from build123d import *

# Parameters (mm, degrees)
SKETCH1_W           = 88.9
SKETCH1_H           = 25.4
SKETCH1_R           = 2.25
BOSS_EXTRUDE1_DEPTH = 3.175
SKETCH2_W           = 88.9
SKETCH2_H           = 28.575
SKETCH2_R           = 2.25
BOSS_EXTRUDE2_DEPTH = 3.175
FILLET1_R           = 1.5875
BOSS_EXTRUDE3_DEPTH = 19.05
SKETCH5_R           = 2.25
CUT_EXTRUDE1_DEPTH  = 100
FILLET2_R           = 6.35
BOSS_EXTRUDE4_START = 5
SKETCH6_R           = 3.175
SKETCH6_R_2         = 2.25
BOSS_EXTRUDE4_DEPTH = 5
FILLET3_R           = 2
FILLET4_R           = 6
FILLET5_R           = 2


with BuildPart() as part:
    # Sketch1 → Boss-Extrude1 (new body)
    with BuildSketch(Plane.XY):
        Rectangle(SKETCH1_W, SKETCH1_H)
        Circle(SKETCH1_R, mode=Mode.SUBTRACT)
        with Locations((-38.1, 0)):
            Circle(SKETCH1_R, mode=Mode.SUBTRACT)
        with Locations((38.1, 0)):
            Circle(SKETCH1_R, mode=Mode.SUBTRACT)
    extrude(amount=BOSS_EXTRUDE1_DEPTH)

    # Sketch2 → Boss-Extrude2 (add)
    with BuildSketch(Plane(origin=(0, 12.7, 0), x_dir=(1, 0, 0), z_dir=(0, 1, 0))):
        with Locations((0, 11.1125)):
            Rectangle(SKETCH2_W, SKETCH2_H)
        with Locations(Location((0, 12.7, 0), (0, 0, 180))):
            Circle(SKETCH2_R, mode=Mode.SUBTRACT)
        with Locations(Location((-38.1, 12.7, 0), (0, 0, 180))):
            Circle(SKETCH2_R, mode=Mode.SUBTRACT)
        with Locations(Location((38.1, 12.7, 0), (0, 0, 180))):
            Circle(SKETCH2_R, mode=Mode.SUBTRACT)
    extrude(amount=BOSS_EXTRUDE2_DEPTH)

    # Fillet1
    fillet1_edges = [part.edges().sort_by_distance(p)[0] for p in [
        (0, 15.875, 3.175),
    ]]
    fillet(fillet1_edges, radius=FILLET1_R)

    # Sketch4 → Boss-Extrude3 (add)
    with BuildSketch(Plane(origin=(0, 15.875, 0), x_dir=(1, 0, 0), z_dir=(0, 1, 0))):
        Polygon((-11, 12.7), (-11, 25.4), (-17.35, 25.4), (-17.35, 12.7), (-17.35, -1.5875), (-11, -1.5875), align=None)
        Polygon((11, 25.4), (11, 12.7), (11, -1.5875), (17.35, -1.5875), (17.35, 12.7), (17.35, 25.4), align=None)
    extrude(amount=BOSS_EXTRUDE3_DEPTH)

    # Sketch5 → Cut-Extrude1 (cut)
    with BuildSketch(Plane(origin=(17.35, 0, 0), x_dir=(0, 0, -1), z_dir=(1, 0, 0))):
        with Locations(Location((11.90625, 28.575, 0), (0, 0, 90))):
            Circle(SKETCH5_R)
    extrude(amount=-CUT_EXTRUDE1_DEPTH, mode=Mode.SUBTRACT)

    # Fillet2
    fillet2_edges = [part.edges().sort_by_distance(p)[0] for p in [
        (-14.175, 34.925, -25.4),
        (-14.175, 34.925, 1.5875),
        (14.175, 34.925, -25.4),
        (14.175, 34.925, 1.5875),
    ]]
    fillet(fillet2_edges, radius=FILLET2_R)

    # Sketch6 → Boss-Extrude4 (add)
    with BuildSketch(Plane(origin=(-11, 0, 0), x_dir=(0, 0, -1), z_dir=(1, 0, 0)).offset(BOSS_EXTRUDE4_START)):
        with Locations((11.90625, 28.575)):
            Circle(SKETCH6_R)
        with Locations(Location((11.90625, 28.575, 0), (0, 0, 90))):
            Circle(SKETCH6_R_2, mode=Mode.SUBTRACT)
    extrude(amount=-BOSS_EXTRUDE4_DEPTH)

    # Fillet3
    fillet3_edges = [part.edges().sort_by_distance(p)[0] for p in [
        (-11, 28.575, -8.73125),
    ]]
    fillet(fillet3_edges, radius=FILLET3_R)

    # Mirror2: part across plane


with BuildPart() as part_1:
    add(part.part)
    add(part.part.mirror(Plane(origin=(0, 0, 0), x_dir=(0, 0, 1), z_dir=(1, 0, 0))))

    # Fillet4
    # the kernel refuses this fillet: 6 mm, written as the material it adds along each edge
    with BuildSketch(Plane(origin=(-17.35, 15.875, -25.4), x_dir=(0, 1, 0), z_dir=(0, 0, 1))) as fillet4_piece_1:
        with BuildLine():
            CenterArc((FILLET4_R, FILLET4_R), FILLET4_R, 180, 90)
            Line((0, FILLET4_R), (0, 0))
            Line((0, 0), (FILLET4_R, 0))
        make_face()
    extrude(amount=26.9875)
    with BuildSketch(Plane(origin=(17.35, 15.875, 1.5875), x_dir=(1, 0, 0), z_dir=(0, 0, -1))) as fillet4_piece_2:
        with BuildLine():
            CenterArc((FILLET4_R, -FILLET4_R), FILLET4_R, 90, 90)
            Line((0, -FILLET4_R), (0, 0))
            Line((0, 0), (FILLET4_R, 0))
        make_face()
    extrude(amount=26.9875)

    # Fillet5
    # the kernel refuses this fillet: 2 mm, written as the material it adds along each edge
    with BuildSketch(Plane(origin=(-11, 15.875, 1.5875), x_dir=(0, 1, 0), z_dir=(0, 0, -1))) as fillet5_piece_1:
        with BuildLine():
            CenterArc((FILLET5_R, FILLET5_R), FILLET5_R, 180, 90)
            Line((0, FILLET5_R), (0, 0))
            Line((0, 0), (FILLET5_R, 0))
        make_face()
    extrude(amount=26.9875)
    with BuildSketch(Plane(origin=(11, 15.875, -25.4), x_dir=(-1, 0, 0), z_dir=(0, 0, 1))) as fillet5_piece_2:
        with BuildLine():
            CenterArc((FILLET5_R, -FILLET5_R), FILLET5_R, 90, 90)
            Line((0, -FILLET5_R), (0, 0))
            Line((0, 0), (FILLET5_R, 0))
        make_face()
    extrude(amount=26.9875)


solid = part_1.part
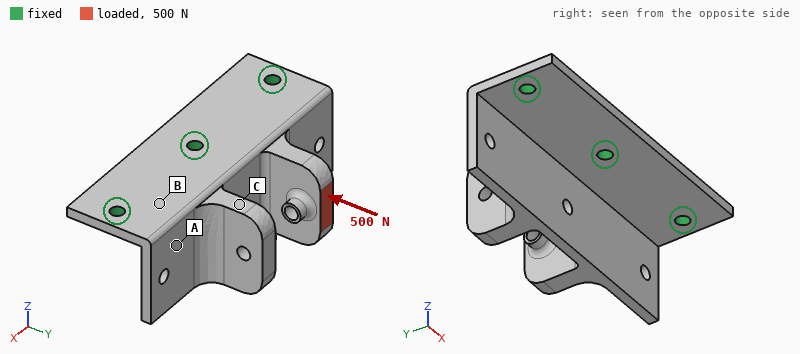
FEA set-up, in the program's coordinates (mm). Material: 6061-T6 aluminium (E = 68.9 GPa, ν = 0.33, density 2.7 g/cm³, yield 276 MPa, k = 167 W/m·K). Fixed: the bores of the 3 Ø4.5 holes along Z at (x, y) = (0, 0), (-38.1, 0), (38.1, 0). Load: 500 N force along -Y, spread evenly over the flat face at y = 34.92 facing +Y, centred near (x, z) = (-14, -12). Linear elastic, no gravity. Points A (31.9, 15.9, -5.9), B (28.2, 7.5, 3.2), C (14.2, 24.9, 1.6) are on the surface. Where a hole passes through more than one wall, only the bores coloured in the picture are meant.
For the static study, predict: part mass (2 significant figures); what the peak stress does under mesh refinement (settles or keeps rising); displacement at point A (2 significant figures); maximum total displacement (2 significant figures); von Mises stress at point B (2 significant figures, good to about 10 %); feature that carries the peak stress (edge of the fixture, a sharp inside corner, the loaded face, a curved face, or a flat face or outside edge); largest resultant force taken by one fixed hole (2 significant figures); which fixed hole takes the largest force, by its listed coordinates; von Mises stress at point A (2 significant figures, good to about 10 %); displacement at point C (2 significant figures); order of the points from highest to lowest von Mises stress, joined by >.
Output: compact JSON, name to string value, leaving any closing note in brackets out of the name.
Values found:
{"part mass": "58 g", "what the peak stress does under mesh refinement": "keeps rising", "displacement at point A": "0.055 mm", "maximum total displacement": "0.30 mm", "von Mises stress at point B": "27 MPa", "feature that carries the peak stress": "edge of the fixture", "largest resultant force taken by one fixed hole": "380 N", "which fixed hole takes the largest force, by its listed coordinates": "(0, 0)", "von Mises stress at point A": "14 MPa", "displacement at point C": "0.10 mm", "order of the points from highest to lowest von Mises stress, joined by >": "B > A > C"}
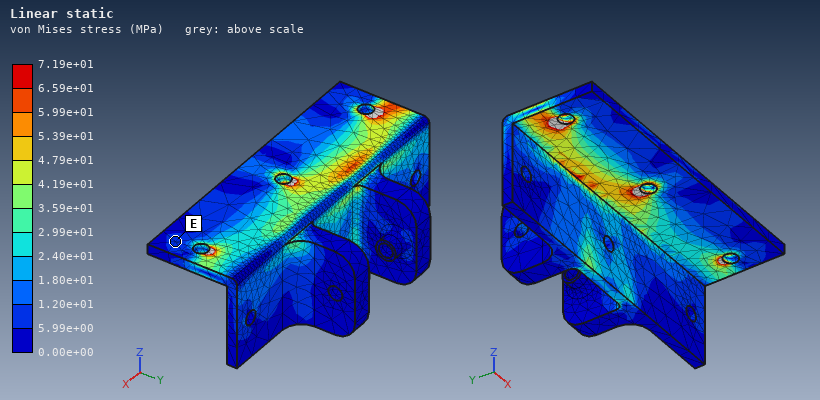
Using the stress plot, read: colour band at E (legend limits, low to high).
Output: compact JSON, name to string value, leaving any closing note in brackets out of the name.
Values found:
{"colour band at E": "5.99e+00 to 1.20e+01 MPa"}
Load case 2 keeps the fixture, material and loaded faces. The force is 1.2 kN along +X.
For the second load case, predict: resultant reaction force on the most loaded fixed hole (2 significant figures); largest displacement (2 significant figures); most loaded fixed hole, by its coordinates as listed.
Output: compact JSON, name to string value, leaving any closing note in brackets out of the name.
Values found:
{"resultant reaction force on the most loaded fixed hole": "1.1 kN", "largest displacement": "0.20 mm", "most loaded fixed hole, by its coordinates as listed": "(-38.1, 0)"}
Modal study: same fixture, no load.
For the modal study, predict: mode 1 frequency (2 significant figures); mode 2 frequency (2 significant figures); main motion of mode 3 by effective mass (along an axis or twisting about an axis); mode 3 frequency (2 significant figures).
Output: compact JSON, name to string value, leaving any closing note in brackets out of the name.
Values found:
{"mode 1 frequency": "1200 Hz", "mode 2 frequency": "2700 Hz", "main motion of mode 3 by effective mass": "along X", "mode 3 frequency": "5100 Hz"}
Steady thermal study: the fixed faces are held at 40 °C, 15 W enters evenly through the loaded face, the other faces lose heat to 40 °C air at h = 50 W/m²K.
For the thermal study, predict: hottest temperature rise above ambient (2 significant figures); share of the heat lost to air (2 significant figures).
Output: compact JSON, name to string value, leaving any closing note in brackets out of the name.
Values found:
{"hottest temperature rise above ambient": "24 K", "share of the heat lost to air": "24 %"}
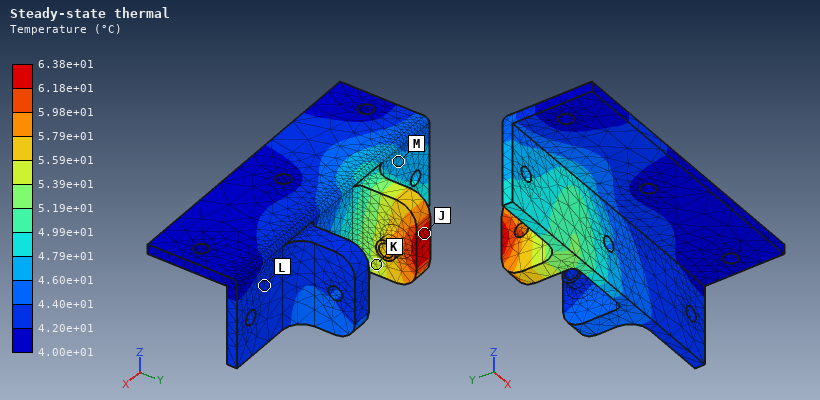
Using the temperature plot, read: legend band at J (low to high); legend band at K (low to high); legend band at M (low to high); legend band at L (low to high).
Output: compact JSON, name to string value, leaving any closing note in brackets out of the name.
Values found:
{"legend band at J": "6.18e+01 to 6.38e+01 °C", "legend band at K": "5.39e+01 to 5.59e+01 °C", "legend band at M": "4.60e+01 to 4.79e+01 °C", "legend band at L": "4.20e+01 to 4.40e+01 °C"}
